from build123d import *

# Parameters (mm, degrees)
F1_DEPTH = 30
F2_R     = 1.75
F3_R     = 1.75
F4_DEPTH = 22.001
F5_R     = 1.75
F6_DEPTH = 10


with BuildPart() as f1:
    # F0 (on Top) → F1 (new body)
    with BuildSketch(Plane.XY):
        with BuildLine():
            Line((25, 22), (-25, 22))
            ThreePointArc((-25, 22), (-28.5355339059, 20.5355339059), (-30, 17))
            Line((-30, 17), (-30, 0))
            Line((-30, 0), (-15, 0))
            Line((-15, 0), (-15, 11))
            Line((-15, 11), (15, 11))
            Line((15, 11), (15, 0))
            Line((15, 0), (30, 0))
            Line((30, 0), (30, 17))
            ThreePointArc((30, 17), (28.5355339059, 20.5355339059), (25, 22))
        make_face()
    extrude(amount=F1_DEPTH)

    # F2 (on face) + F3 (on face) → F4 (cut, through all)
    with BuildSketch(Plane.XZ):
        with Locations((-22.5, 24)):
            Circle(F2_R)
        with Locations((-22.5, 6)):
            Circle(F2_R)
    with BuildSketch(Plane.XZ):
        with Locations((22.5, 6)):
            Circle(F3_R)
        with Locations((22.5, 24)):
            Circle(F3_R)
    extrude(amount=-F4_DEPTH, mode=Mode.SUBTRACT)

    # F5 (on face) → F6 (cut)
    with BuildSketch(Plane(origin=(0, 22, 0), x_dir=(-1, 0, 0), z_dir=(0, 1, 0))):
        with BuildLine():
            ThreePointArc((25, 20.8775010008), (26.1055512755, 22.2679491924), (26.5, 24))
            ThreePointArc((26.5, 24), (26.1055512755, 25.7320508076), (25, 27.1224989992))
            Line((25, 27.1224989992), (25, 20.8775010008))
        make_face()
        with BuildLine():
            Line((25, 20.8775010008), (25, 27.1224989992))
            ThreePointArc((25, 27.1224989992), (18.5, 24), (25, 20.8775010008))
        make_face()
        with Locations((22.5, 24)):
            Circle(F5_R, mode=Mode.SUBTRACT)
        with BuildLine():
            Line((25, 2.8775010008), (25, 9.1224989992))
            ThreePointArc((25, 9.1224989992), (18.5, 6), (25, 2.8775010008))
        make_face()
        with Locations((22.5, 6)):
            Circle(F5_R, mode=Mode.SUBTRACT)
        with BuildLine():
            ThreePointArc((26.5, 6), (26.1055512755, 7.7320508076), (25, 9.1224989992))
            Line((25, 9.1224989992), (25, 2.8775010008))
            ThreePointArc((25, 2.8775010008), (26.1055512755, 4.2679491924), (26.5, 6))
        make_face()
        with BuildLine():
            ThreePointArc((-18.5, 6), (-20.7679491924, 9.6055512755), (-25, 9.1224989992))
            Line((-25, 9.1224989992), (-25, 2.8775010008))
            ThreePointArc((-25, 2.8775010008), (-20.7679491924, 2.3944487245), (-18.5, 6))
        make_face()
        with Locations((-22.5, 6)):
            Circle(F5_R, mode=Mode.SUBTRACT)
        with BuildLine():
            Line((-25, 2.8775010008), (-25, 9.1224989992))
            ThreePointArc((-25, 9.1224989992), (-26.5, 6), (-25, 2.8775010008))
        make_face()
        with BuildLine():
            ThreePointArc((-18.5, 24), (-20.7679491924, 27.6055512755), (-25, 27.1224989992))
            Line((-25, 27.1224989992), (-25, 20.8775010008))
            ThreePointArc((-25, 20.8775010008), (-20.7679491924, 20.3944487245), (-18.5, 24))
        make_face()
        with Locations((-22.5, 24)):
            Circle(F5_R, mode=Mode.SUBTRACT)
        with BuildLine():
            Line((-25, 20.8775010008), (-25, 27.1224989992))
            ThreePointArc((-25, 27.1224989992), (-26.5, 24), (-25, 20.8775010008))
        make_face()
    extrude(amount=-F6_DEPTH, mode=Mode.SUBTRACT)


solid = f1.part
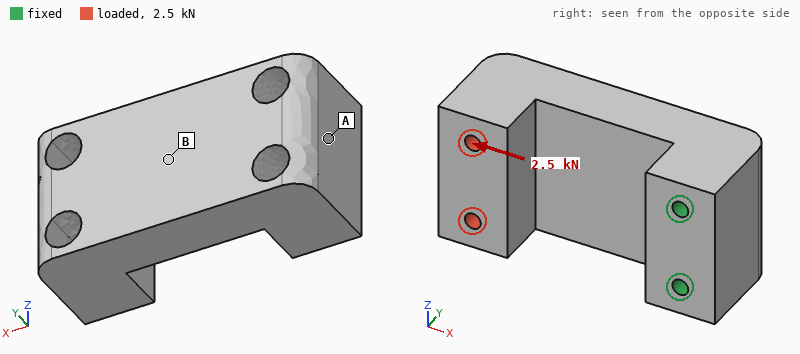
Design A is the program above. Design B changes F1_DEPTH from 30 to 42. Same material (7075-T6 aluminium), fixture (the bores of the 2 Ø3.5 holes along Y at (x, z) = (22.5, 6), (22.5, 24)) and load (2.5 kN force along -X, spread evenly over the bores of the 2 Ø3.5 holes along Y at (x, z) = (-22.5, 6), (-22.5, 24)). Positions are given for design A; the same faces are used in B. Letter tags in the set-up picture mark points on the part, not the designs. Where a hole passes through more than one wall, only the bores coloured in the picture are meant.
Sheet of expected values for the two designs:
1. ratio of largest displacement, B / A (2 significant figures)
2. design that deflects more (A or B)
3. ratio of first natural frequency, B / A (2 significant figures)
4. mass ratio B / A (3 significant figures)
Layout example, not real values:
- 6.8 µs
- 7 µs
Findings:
- 0.73
- A
- 0.95
- 1.44
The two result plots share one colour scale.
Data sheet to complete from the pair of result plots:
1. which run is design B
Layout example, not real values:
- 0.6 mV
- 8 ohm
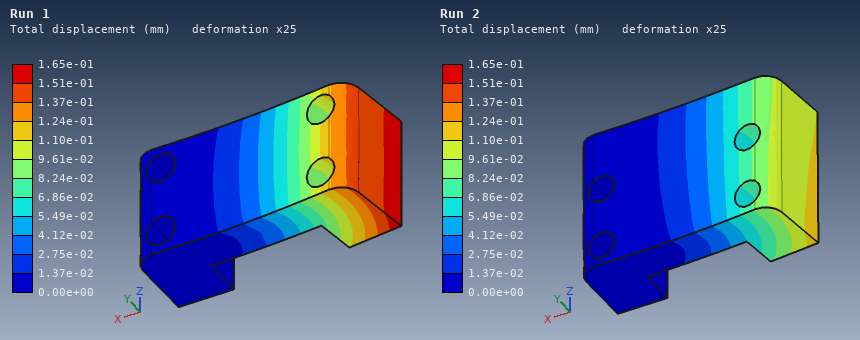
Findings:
- Run 2
